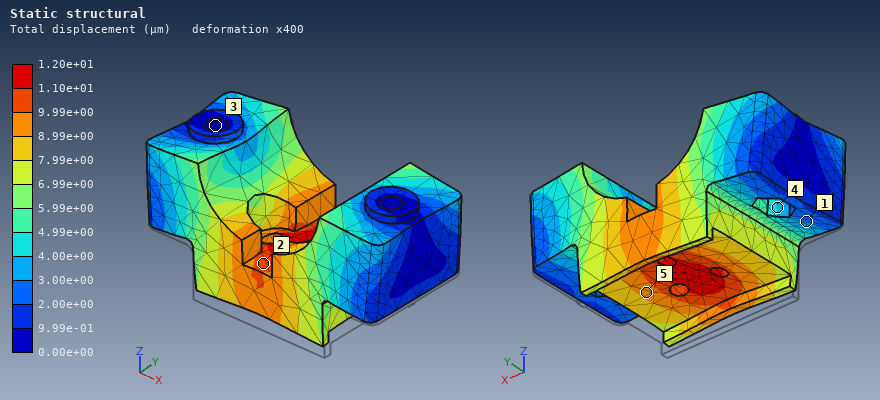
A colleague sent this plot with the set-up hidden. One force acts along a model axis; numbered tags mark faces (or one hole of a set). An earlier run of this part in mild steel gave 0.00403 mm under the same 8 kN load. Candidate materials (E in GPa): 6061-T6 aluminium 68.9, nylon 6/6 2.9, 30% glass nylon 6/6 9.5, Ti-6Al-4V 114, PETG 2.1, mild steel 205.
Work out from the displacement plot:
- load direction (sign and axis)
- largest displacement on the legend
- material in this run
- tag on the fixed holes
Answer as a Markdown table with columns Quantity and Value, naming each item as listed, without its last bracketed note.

| Quantity | Value |
|---|---|
| load direction | +Z |
| largest displacement on the legend | 1.20e+01 µm |
| material in this run | 6061-T6 aluminium |
| tag on the fixed holes | 3 |
